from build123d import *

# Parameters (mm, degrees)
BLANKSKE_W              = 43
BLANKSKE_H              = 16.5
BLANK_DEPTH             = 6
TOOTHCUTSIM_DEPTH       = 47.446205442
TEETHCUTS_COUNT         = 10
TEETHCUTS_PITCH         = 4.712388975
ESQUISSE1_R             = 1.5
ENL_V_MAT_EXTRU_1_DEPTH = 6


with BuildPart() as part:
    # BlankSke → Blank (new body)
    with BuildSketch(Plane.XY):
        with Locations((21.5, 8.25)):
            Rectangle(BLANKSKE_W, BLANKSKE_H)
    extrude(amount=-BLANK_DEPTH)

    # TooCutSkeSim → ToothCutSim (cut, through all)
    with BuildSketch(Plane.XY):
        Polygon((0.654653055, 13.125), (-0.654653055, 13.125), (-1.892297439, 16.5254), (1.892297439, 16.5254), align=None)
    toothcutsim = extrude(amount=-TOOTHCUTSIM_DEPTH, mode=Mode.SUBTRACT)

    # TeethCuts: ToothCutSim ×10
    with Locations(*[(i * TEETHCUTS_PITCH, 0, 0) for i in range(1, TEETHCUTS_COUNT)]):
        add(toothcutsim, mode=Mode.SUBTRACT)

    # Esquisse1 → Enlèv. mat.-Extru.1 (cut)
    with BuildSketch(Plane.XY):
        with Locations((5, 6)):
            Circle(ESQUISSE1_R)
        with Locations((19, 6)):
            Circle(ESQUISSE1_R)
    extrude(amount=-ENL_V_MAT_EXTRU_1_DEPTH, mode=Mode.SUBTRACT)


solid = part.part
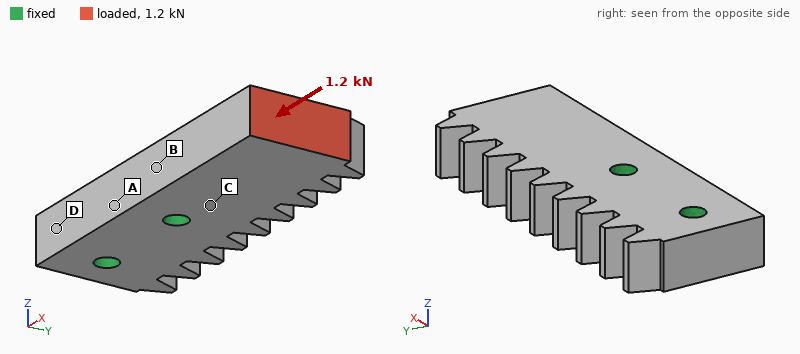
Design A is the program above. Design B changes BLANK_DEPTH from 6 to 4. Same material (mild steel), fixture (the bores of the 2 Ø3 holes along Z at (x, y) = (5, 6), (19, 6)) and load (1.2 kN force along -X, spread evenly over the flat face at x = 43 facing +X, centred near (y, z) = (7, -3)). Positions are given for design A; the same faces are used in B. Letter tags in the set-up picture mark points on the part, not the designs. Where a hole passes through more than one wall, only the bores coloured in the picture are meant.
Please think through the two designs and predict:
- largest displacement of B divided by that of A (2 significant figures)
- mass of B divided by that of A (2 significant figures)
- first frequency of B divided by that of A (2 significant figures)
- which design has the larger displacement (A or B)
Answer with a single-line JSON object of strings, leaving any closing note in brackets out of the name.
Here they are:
{"largest displacement of B divided by that of A": "1.5", "mass of B divided by that of A": "0.67", "first frequency of B divided by that of A": "0.70", "which design has the larger displacement": "B"}
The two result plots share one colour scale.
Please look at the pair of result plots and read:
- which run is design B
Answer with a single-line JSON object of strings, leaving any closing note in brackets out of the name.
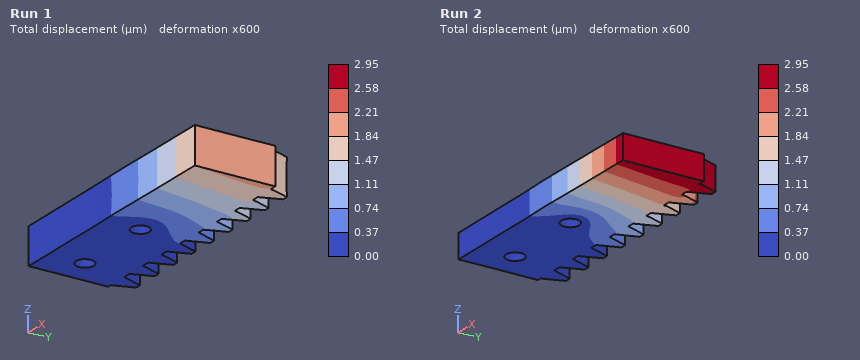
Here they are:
{"which run is design B": "Run 2"}
